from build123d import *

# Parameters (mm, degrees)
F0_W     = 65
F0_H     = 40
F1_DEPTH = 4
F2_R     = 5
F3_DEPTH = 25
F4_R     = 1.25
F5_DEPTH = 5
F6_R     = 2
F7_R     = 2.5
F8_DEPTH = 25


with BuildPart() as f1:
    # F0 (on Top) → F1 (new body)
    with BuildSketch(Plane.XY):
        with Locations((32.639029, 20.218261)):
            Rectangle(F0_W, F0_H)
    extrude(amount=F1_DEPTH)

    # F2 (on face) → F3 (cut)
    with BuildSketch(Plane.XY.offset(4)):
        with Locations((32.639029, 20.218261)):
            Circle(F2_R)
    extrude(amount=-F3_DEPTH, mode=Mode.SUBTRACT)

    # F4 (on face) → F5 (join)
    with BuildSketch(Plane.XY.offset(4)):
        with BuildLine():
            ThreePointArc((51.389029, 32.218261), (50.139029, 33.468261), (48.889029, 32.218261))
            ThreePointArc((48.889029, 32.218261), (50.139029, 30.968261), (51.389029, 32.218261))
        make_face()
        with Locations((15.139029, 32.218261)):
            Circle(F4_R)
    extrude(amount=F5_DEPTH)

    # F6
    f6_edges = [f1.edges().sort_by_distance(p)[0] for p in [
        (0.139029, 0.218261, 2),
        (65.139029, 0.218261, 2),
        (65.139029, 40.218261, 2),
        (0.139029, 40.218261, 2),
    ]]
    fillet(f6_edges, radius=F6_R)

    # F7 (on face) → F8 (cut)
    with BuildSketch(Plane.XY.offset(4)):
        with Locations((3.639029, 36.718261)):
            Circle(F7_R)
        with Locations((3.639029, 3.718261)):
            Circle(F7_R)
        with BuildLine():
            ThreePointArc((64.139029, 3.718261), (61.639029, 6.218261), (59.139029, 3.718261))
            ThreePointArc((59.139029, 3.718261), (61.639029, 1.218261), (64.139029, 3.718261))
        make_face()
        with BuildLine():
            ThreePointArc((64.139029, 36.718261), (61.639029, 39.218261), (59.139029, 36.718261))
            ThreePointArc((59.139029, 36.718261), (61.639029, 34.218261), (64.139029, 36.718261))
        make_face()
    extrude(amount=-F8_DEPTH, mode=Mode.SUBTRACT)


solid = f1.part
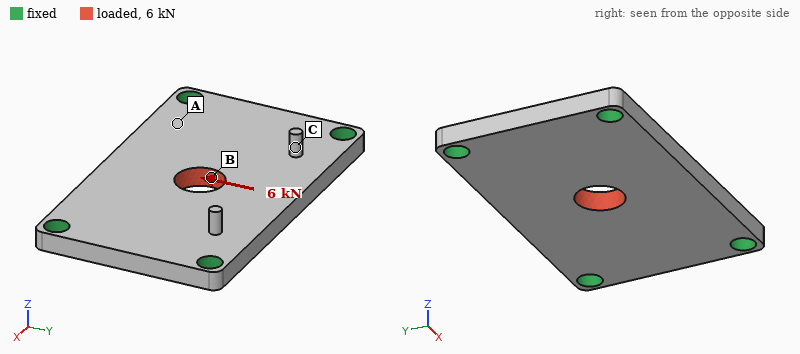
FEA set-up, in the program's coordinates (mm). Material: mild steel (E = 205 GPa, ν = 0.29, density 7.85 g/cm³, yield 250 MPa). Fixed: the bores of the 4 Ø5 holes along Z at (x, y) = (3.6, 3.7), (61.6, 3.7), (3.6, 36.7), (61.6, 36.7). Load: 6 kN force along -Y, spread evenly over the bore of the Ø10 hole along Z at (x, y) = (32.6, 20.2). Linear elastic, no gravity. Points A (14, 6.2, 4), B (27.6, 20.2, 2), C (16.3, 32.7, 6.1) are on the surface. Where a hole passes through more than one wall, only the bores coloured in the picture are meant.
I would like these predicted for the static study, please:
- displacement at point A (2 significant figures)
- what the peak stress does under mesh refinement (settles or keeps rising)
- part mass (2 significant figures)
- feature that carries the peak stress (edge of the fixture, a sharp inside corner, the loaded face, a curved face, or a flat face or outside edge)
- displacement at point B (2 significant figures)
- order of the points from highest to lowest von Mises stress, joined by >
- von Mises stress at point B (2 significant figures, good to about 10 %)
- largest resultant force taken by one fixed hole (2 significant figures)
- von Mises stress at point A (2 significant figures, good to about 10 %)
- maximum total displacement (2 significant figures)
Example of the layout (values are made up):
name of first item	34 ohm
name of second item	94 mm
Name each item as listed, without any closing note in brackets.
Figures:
displacement at point A	3.3 µm
what the peak stress does under mesh refinement	keeps rising
part mass	77 g
feature that carries the peak stress	edge of the fixture
displacement at point B	8.5 µm
order of the points from highest to lowest von Mises stress, joined by >	B > A > C
von Mises stress at point B	84 MPa
largest resultant force taken by one fixed hole	2.0 kN
von Mises stress at point A	34 MPa
maximum total displacement	9.2 µm
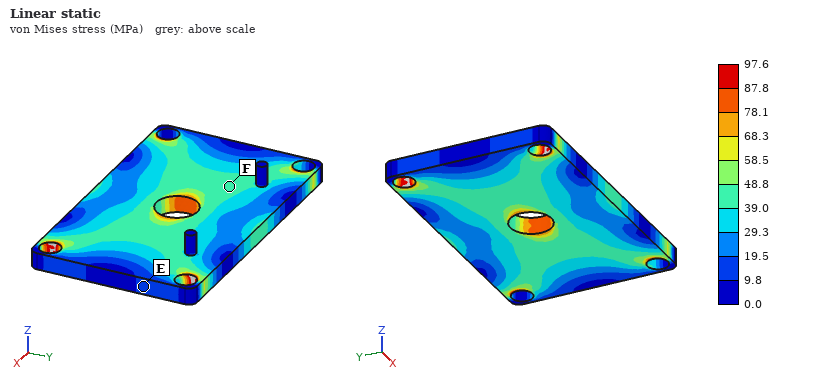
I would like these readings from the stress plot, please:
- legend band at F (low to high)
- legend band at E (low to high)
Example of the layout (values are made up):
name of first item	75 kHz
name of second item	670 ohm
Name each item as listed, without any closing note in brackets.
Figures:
legend band at F	39.0 to 48.8 MPa
legend band at E	9.8 to 19.5 MPa
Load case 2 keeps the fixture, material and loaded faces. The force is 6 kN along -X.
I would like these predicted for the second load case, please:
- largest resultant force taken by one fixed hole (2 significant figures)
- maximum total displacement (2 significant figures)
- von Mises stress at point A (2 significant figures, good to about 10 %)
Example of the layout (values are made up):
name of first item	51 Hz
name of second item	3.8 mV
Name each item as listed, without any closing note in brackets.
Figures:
largest resultant force taken by one fixed hole	1.6 kN
maximum total displacement	4.8 µm
von Mises stress at point A	28 MPa
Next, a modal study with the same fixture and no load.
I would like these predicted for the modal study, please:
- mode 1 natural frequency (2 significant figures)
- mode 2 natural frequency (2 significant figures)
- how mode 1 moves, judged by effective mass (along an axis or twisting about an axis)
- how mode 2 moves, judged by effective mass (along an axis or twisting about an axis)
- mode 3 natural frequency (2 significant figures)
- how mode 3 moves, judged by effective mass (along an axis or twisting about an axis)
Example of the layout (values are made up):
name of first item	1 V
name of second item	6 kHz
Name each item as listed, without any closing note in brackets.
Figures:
mode 1 natural frequency	5700 Hz
mode 2 natural frequency	8900 Hz
how mode 1 moves, judged by effective mass	along Z
how mode 2 moves, judged by effective mass	twisting about X
mode 3 natural frequency	14 kHz
how mode 3 moves, judged by effective mass	twisting about Y
